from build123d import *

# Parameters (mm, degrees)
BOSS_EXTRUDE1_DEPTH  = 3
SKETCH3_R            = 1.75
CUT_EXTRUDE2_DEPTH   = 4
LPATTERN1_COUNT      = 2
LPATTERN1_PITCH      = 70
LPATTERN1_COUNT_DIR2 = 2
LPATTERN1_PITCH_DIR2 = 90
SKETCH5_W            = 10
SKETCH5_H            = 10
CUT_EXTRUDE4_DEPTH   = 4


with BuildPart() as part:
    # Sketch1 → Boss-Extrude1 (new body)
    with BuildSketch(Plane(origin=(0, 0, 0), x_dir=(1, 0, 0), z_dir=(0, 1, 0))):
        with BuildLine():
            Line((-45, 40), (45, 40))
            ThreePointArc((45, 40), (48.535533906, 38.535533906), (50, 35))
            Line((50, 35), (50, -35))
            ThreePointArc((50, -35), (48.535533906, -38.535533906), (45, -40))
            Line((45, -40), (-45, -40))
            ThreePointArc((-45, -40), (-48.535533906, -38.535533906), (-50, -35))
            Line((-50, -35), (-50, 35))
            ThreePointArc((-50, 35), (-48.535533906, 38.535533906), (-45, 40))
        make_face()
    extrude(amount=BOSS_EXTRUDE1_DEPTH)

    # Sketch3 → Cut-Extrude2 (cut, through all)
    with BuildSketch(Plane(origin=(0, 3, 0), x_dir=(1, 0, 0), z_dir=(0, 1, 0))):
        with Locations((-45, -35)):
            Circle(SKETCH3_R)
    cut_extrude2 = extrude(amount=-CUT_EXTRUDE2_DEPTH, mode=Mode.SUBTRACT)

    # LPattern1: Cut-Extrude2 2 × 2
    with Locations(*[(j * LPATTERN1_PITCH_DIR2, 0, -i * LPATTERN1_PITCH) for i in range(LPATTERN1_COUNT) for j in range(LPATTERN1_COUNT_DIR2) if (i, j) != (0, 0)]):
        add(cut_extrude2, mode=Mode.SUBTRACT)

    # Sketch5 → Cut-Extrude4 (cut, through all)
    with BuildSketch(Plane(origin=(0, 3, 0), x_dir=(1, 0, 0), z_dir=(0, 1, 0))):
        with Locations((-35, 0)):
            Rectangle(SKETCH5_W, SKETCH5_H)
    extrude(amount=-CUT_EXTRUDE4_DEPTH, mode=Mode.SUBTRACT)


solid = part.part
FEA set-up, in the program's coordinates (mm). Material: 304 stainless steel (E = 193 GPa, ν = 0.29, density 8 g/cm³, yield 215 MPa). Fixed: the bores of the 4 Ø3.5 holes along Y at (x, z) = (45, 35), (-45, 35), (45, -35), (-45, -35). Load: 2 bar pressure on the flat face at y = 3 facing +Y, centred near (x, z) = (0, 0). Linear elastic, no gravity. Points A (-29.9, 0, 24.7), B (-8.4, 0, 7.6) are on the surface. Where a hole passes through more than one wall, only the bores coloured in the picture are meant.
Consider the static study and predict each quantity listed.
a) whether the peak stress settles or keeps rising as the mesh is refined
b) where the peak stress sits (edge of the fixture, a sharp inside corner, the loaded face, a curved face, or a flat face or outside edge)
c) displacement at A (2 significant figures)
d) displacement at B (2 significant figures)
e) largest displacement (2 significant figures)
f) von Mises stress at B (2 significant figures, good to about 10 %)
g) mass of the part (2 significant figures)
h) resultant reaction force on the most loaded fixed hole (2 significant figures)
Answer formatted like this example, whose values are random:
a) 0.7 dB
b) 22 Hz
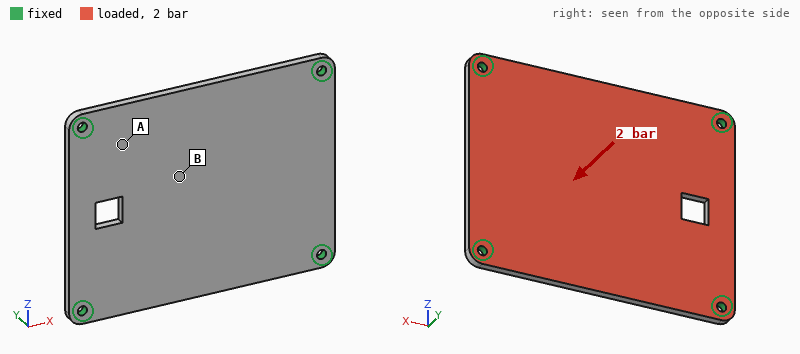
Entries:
a) keeps rising
b) edge of the fixture
c) 0.064 mm
d) 0.15 mm
e) 0.16 mm
f) 48 MPa
g) 190 g
h) 400 N
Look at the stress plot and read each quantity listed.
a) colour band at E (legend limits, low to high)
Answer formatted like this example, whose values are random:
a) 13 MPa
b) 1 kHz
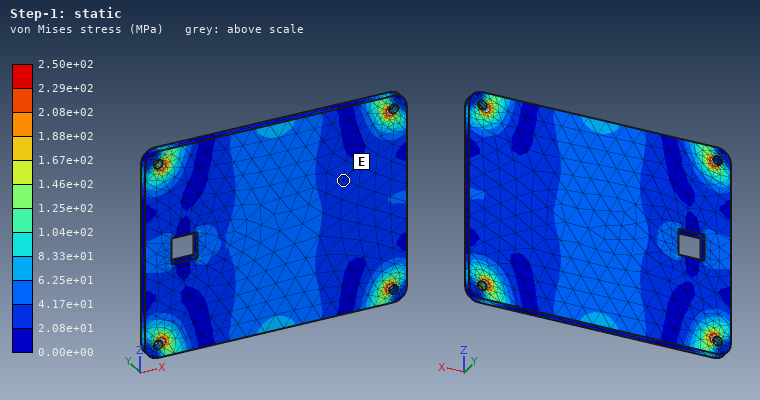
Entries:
a) 2.08e+01 to 4.17e+01 MPa
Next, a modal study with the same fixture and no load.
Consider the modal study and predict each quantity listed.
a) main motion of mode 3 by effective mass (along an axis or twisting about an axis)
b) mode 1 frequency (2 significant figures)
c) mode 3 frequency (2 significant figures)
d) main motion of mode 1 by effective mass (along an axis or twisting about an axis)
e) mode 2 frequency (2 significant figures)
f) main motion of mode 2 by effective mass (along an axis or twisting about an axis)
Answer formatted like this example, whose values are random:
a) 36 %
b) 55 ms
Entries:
a) twisting about Z
b) 1400 Hz
c) 3000 Hz
d) along Y
e) 2300 Hz
f) twisting about X
